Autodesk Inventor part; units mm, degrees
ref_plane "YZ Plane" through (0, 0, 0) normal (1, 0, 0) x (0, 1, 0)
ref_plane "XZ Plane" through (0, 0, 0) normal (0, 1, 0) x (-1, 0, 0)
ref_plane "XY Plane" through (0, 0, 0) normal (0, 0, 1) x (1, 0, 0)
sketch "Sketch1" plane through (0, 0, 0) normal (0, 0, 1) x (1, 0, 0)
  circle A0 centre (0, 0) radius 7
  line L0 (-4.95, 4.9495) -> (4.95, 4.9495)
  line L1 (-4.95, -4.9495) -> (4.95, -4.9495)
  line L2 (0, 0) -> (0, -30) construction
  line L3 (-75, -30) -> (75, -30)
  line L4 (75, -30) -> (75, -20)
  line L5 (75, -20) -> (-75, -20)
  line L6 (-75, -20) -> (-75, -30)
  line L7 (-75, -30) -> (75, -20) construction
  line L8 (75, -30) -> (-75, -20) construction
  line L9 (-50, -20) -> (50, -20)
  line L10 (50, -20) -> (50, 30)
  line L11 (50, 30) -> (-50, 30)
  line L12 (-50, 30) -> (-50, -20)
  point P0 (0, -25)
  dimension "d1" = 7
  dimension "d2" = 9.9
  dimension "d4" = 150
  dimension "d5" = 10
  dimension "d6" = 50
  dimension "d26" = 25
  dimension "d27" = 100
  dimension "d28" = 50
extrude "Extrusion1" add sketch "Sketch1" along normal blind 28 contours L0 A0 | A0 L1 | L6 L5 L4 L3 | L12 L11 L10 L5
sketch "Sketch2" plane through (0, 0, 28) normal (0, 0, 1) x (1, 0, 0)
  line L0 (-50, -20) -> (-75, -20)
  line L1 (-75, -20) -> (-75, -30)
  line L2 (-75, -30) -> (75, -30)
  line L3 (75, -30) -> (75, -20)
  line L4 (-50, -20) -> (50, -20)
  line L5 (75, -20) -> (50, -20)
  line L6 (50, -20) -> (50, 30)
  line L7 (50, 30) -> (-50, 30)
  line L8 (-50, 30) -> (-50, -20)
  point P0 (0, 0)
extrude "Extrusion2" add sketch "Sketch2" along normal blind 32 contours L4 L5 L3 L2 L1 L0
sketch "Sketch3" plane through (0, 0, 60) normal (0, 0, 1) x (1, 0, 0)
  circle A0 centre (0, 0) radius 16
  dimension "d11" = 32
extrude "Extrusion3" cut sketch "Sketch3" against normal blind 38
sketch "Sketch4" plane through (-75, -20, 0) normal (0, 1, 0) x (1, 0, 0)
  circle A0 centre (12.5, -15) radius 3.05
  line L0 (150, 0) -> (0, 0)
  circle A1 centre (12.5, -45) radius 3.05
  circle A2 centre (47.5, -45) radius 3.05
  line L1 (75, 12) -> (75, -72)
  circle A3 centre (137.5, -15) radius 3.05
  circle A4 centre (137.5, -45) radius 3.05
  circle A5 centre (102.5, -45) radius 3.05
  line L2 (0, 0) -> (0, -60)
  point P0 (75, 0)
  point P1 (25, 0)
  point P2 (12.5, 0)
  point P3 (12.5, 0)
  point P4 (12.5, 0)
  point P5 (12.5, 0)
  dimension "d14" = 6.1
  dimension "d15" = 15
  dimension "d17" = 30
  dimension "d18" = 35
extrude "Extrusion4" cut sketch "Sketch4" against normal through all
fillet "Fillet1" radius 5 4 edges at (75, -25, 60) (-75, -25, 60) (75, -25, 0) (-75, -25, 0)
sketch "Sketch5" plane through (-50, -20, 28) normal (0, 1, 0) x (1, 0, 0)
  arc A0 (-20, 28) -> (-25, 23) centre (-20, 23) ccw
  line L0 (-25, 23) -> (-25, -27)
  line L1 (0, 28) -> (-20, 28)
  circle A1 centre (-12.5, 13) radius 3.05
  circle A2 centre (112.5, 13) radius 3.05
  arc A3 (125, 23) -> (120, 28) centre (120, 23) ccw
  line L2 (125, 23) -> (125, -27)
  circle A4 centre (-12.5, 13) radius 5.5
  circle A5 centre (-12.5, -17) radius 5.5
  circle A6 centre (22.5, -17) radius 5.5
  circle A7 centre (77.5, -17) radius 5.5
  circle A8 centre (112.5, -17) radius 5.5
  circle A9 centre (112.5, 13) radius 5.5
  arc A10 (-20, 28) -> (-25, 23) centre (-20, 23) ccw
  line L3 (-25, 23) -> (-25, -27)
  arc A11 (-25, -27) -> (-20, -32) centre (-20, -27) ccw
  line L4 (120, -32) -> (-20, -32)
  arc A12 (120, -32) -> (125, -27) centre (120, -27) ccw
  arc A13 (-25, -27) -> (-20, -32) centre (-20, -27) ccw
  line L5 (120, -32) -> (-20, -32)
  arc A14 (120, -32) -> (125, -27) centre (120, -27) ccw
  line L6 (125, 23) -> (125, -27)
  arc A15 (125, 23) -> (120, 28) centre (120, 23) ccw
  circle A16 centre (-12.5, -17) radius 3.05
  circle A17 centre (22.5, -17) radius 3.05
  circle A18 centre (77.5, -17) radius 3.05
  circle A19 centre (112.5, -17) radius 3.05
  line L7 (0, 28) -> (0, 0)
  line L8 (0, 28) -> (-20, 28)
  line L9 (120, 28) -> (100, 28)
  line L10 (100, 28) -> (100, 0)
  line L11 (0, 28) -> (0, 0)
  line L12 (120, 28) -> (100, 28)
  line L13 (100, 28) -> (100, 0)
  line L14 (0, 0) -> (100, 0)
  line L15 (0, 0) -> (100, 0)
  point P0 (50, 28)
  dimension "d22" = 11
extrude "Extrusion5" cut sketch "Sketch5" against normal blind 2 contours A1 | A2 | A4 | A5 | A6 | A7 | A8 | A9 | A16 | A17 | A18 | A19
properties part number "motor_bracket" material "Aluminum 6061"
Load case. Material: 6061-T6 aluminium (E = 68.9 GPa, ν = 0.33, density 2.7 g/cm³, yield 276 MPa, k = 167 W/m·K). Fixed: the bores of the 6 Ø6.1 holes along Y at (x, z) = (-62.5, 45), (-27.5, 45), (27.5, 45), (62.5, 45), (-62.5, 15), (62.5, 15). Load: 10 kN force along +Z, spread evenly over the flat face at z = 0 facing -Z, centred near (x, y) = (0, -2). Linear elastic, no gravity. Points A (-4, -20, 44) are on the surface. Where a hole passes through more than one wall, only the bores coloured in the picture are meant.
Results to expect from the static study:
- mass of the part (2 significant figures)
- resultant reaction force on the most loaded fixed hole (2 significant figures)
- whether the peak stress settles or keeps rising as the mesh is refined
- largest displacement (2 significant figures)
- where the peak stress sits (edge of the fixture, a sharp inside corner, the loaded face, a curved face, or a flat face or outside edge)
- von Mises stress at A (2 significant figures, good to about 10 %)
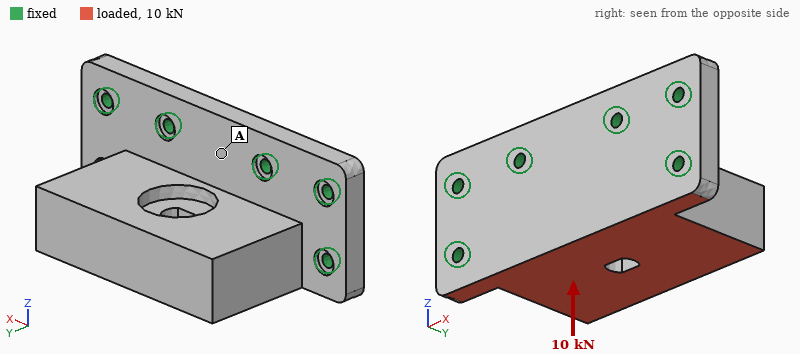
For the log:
590 g
4.5 kN
keeps rising
0.15 mm
edge of the fixture
15 MPa
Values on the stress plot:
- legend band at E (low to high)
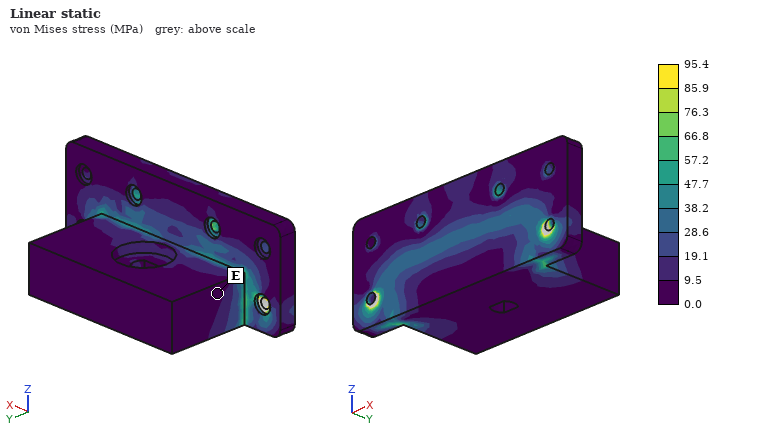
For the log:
0.0 to 9.5 MPa
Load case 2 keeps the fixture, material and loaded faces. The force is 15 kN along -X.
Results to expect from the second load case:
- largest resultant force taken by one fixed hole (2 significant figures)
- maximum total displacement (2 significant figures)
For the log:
5.2 kN
32 µm
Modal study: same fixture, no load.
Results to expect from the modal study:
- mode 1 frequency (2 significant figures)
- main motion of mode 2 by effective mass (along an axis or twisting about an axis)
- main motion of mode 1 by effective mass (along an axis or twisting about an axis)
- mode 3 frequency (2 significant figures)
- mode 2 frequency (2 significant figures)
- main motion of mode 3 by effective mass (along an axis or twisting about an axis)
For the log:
2200 Hz
along X
along Z
5800 Hz
5500 Hz
along Y
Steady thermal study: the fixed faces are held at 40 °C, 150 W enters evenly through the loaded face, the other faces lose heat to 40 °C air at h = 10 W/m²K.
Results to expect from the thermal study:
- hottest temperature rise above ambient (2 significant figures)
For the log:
24 K
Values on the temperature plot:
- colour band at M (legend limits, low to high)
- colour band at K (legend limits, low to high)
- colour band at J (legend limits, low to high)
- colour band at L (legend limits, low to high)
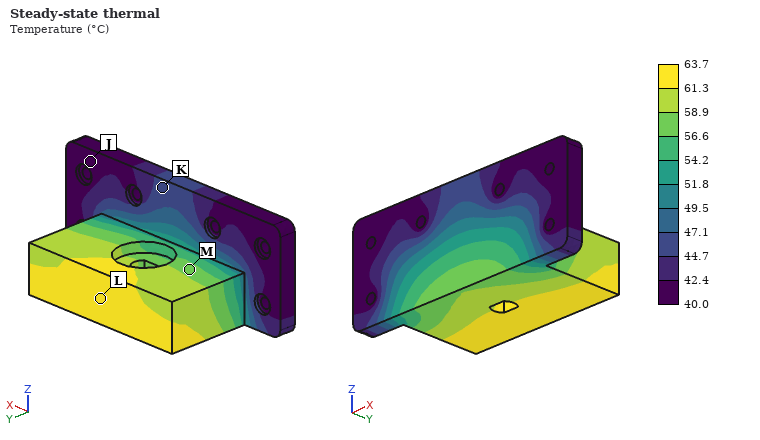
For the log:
56.6 to 58.9 °C
44.7 to 47.1 °C
40.0 to 42.4 °C
61.3 to 63.7 °C
